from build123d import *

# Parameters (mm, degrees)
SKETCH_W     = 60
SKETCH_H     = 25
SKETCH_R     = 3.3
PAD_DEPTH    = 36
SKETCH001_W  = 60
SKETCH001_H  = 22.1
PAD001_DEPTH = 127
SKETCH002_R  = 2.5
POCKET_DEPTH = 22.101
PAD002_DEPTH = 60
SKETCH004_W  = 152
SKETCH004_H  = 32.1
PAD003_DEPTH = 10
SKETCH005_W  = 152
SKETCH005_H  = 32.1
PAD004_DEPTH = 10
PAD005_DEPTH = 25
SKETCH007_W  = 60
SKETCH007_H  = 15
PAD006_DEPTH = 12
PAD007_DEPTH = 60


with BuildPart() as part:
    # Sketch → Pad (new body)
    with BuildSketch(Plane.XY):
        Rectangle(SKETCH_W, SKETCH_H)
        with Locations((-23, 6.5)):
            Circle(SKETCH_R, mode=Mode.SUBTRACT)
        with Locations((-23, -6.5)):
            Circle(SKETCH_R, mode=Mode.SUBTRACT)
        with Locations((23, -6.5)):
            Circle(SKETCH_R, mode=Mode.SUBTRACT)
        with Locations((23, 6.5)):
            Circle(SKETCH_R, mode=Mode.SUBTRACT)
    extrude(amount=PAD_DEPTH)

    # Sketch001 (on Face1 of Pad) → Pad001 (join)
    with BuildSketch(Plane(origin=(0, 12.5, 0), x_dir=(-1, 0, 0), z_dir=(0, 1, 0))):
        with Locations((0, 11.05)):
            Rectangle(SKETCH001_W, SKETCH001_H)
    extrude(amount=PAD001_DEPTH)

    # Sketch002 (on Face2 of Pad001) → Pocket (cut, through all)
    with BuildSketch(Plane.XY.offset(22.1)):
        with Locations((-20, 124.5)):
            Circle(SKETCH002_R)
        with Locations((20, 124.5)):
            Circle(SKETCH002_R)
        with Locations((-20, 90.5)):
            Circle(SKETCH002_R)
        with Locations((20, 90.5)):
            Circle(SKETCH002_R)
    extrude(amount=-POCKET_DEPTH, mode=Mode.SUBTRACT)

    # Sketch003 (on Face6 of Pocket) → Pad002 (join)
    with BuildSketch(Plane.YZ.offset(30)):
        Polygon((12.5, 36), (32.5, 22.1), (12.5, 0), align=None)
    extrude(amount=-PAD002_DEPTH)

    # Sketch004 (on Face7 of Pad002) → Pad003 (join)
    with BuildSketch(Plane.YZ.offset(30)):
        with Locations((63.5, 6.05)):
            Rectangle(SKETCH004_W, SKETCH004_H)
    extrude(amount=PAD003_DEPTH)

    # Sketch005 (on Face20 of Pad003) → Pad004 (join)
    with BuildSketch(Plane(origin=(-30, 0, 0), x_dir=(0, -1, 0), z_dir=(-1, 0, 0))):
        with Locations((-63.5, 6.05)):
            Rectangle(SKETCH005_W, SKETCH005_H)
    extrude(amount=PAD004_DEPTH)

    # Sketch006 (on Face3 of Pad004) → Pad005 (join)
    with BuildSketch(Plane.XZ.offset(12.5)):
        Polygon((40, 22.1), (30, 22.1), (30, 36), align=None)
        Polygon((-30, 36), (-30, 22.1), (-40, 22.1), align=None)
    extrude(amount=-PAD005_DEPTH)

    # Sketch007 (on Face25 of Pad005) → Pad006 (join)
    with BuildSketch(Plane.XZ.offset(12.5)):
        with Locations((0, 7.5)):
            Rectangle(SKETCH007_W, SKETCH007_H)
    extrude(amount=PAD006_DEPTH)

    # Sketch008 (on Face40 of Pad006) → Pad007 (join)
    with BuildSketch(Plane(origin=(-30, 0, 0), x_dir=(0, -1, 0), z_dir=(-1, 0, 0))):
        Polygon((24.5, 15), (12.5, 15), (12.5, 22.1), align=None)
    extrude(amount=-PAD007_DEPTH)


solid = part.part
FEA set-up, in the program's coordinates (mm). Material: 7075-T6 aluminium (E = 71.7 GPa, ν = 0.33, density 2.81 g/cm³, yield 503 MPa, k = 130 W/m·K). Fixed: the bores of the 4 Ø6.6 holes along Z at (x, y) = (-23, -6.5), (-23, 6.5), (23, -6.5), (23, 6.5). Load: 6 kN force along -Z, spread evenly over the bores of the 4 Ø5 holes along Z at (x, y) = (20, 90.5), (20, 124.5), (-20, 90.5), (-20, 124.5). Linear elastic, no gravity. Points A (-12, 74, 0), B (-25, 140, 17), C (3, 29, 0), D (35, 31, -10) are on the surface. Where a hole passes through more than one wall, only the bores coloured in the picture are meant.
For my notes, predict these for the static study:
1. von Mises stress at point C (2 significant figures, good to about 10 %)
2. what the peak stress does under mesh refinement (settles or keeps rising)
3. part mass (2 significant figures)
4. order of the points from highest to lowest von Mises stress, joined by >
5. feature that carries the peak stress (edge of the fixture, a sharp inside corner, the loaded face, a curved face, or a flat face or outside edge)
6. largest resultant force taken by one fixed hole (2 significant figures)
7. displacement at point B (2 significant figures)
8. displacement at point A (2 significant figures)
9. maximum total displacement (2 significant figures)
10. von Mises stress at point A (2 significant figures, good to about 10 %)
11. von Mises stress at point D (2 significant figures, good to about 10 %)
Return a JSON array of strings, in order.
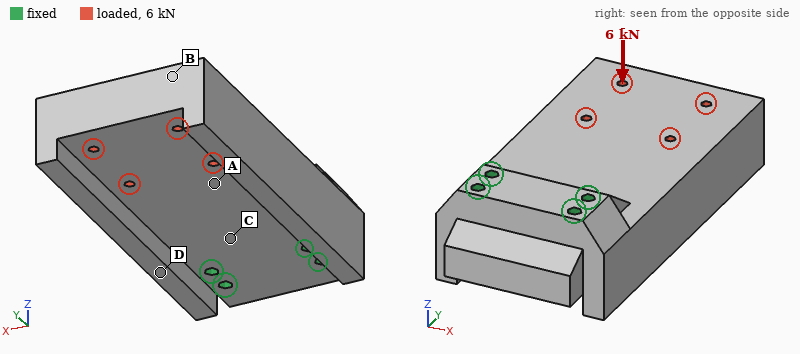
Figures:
["37 MPa", "keeps rising", "950 g", "D > C > A > B", "edge of the fixture", "6.1 kN", "0.32 mm", "0.12 mm", "0.33 mm", "15 MPa", "57 MPa"]
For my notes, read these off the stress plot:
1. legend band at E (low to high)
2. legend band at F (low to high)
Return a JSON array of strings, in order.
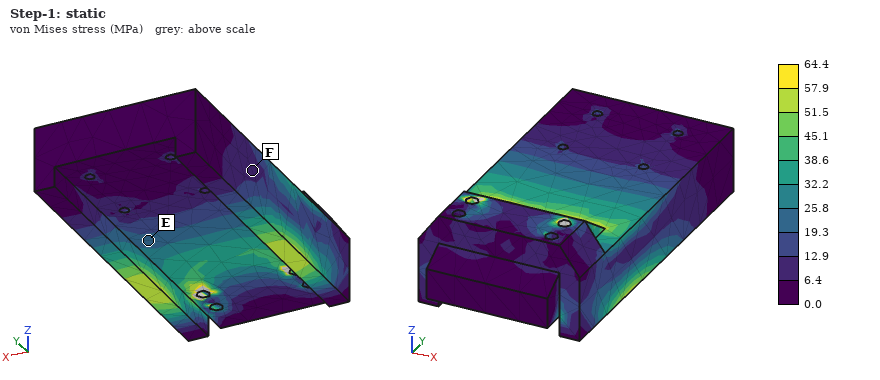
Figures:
["19.3 to 25.8 MPa", "6.4 to 12.9 MPa"]
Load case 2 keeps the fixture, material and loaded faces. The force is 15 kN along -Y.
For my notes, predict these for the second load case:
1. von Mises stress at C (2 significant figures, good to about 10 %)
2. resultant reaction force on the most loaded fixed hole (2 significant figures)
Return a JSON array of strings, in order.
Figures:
["5.6 MPa", "5.6 kN"]
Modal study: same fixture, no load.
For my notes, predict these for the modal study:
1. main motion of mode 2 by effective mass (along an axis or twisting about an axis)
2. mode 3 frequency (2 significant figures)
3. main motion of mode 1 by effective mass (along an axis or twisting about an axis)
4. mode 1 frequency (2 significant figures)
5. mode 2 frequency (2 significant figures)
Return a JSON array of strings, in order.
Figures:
["along X", "3200 Hz", "along Z", "1300 Hz", "2800 Hz"]
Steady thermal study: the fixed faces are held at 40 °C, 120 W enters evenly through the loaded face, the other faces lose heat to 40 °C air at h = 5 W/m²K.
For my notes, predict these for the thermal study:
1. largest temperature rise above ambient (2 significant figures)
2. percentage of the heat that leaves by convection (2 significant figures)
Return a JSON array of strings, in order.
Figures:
["48 K", "4.1 %"]
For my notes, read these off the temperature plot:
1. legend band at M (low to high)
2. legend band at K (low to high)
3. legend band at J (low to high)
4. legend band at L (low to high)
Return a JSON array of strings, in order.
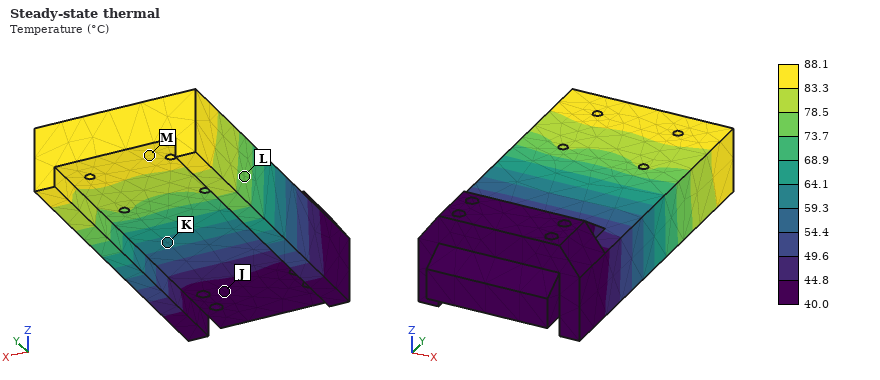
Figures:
["83.3 to 88.1 °C", "59.3 to 64.1 °C", "40.0 to 44.8 °C", "73.7 to 78.5 °C"]
